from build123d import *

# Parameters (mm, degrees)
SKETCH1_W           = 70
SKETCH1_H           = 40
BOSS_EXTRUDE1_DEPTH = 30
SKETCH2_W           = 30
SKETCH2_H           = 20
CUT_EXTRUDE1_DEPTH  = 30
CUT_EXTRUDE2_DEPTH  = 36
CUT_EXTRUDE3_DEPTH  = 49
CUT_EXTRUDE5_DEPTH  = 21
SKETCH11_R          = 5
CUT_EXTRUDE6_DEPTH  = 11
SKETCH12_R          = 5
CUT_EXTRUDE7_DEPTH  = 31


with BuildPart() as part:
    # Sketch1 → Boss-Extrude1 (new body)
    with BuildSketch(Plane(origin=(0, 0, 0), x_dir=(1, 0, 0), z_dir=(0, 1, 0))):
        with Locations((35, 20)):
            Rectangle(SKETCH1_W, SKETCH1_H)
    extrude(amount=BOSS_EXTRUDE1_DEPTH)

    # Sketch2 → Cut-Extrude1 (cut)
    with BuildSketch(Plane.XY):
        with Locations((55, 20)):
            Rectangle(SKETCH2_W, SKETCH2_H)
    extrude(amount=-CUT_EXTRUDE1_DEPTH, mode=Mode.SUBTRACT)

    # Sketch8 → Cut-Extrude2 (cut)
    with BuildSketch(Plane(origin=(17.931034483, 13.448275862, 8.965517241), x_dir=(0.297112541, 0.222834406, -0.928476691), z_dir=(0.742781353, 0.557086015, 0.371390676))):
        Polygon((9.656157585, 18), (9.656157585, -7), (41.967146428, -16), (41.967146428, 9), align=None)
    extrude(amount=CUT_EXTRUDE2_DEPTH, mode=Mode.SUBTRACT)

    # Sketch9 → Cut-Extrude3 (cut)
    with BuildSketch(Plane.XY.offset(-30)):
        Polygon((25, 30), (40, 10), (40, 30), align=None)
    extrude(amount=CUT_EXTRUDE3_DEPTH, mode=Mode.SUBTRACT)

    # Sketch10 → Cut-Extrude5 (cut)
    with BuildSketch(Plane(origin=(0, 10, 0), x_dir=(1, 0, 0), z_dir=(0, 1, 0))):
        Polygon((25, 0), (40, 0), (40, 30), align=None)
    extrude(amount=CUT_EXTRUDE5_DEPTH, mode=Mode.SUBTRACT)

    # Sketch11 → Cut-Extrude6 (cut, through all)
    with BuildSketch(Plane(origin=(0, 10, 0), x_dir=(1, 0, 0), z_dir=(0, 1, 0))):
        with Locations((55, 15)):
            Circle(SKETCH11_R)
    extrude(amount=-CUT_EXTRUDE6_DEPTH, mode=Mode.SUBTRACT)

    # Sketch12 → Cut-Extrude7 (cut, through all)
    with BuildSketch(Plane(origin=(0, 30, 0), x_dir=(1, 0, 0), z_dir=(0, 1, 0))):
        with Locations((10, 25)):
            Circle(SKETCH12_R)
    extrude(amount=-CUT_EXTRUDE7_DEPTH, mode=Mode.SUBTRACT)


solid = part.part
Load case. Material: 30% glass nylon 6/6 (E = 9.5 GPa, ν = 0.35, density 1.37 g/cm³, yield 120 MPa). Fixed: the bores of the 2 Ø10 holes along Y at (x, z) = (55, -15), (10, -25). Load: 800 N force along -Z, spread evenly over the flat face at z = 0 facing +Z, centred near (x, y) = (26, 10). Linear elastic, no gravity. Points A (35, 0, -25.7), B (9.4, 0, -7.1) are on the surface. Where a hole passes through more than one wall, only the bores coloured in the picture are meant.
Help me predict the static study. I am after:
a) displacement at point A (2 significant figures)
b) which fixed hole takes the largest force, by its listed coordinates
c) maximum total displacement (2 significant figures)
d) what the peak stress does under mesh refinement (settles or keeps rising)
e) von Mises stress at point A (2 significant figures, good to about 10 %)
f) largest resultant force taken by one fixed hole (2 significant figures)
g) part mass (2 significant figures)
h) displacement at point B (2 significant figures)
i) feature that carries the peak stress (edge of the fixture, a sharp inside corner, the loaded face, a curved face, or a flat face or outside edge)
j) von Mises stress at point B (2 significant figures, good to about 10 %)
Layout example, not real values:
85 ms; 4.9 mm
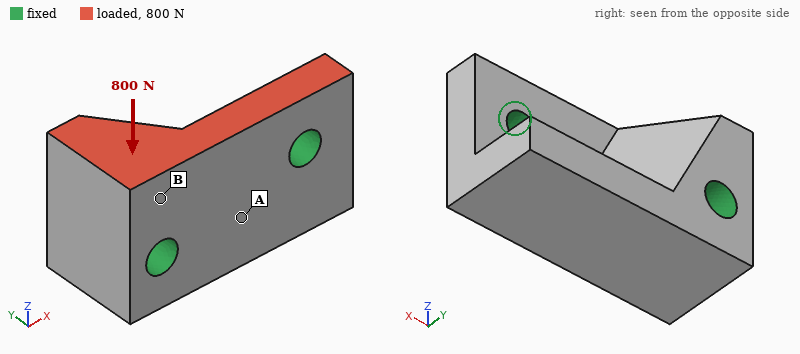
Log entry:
1.3 µm; (10, -25); 3.0 µm; keeps rising; 0.28 MPa; 520 N; 74 g; 1.8 µm; edge of the fixture; 0.87 MPa
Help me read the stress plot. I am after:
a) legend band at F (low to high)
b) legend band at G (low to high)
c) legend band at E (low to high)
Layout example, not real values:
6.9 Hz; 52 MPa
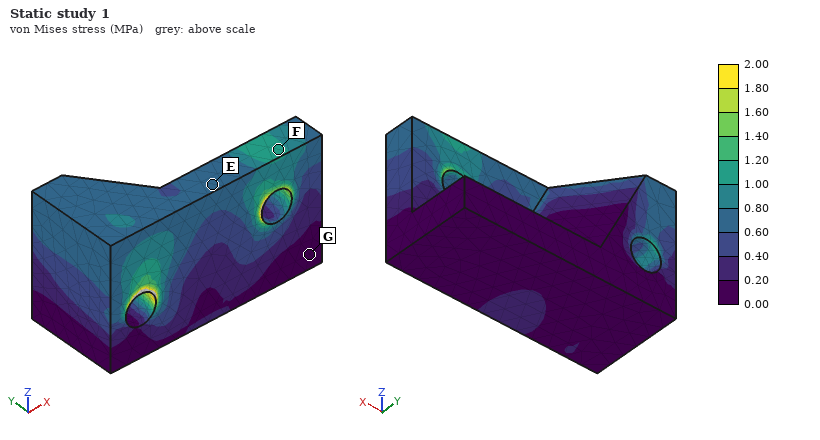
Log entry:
1.00 to 1.20 MPa; 0.00 to 0.20 MPa; 0.60 to 0.80 MPa
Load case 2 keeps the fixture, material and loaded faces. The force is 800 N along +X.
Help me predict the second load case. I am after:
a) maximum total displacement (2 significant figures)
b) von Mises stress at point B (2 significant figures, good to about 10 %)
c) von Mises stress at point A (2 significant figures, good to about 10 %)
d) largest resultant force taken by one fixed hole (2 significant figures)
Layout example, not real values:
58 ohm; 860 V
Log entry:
11 µm; 1.1 MPa; 0.48 MPa; 470 N
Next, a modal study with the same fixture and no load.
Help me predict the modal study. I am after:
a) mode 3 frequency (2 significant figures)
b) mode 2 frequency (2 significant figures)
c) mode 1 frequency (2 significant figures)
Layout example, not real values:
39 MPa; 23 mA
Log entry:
11 kHz; 8300 Hz; 5100 Hz
